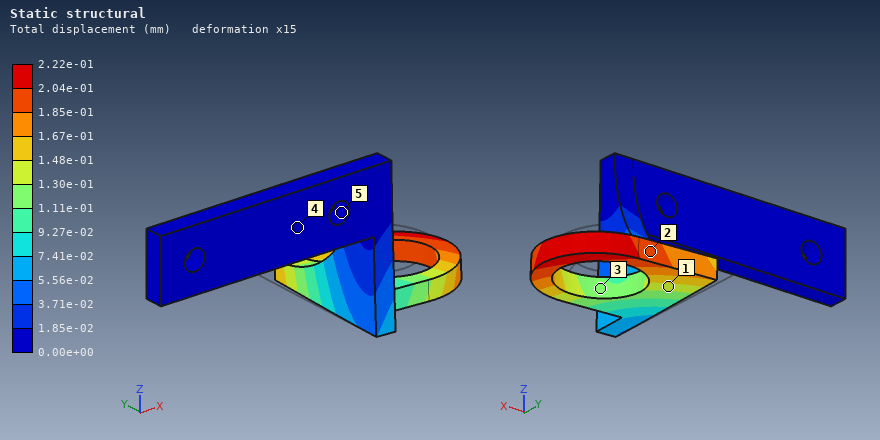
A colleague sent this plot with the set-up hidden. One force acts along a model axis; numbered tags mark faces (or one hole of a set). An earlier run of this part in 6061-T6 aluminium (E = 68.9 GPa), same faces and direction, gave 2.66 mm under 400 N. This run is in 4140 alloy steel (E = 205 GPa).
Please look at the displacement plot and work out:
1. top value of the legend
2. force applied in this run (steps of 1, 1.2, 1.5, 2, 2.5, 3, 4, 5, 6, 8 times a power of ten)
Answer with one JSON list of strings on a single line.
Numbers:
["2.22e-01 mm", "100 N"]
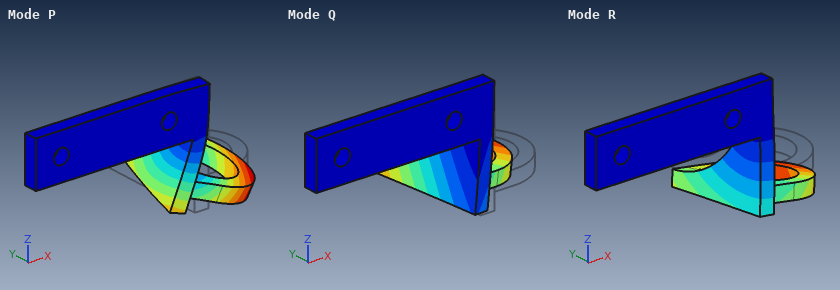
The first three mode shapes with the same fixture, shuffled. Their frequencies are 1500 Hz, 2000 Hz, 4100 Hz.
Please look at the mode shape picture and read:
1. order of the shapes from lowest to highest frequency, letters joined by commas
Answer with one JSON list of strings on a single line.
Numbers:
["Q, R, P"]
